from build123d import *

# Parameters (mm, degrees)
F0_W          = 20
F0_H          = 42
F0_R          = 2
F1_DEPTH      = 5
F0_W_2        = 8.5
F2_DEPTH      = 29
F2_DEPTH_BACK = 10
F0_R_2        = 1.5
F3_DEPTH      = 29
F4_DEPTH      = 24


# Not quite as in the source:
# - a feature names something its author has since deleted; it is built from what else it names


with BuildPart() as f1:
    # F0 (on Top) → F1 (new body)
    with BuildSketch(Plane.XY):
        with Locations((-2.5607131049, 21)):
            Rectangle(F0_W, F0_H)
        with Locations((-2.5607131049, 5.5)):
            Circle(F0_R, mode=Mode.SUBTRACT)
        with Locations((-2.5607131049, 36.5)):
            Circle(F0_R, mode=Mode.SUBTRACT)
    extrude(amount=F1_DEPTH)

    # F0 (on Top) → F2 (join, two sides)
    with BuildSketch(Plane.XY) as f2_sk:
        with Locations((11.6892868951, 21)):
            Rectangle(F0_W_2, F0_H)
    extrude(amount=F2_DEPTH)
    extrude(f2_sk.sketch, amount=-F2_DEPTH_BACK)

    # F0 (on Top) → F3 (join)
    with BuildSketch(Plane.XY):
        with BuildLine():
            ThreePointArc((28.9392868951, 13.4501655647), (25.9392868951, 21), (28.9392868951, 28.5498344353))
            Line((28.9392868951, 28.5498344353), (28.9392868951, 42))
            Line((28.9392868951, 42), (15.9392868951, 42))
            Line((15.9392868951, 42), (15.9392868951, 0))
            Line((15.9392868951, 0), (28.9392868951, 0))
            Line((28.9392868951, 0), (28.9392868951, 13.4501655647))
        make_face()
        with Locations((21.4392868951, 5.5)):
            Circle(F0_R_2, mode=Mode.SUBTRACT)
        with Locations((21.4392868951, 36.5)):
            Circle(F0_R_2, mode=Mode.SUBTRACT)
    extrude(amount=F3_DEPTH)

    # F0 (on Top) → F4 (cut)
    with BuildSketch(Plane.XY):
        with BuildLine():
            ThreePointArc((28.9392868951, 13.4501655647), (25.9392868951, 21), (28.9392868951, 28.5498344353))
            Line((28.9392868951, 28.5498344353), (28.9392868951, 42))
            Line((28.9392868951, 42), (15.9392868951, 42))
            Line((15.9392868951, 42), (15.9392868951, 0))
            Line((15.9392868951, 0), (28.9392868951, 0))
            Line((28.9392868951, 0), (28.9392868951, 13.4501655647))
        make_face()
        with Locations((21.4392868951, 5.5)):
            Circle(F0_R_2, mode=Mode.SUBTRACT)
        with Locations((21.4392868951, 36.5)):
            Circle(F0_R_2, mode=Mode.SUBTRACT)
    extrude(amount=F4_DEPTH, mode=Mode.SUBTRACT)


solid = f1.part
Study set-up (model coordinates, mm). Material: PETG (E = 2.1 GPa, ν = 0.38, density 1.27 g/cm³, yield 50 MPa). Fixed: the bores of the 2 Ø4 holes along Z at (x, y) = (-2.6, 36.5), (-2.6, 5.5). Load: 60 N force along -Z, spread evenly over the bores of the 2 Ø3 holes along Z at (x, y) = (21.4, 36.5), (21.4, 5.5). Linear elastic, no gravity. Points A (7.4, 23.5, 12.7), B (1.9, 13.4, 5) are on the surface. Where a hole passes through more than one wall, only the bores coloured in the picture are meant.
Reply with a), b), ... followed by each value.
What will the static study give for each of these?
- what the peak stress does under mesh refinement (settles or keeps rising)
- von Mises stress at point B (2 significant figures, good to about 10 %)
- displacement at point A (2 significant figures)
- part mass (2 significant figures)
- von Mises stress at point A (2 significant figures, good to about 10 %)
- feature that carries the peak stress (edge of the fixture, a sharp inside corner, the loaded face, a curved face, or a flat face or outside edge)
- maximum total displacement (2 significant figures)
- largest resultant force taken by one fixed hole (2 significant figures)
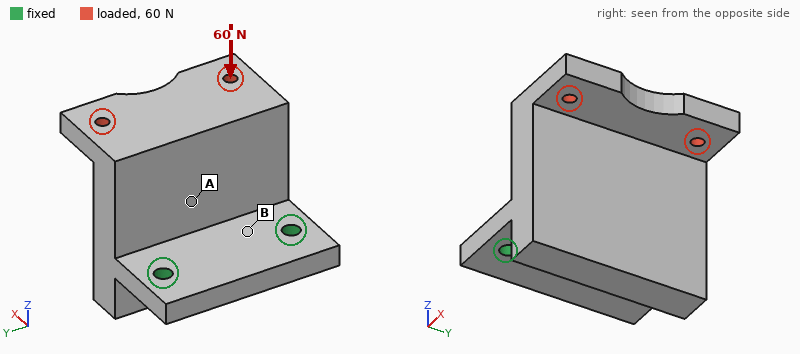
a) keeps rising
b) 4.5 MPa
c) 0.17 mm
d) 26 g
e) 1.0 MPa
f) edge of the fixture
g) 0.64 mm
h) 30 N
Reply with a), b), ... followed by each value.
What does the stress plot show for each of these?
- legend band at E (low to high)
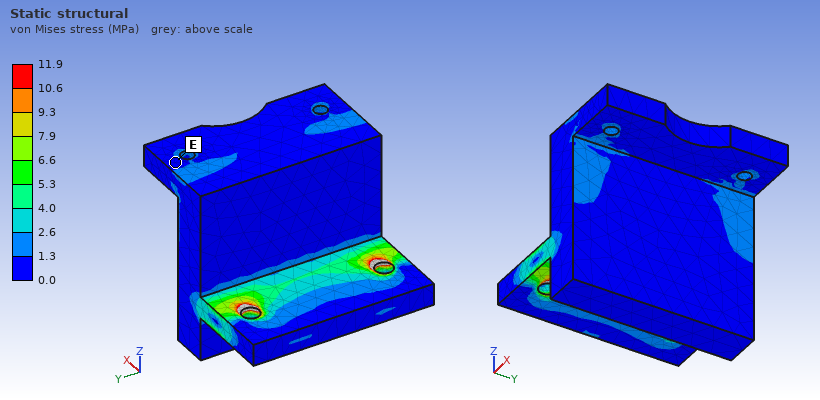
a) 0.0 to 1.3 MPa
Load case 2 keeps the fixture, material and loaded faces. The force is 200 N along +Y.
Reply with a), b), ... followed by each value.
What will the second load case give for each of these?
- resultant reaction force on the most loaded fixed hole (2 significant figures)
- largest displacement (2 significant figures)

a) 230 N
b) 0.30 mm
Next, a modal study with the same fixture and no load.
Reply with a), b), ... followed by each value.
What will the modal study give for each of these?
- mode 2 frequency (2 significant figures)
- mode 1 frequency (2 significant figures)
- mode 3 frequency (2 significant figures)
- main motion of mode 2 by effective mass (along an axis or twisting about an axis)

a) 1400 Hz
b) 490 Hz
c) 2200 Hz
d) along Y
